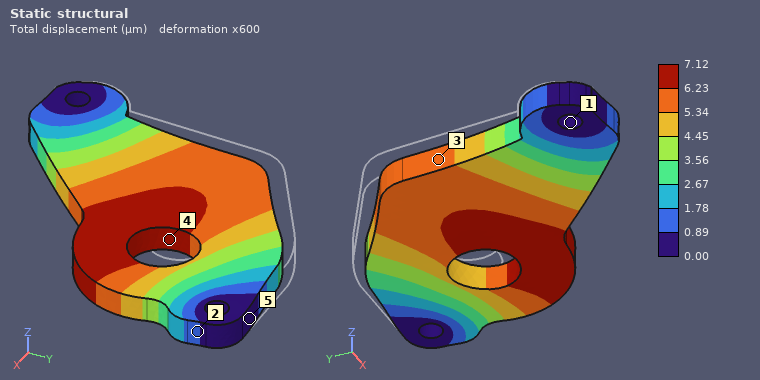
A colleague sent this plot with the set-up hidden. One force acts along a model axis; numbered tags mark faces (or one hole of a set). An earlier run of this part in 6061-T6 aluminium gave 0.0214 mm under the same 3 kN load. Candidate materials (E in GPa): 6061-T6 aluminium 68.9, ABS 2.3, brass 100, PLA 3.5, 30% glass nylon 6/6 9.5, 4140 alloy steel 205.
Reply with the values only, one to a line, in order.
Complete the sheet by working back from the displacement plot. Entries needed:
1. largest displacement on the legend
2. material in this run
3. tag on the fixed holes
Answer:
7.12 µm
4140 alloy steel
1
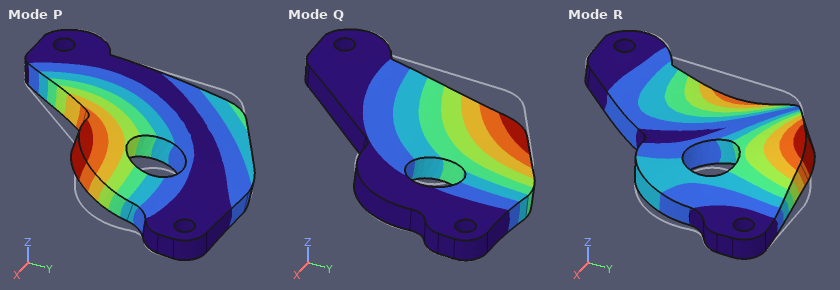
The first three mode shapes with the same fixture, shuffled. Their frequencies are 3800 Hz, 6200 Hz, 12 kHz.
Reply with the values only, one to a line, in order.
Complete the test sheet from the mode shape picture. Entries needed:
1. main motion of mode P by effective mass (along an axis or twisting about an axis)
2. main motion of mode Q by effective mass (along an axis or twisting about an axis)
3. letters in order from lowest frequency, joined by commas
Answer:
along Z
along Z
Q, P, R
